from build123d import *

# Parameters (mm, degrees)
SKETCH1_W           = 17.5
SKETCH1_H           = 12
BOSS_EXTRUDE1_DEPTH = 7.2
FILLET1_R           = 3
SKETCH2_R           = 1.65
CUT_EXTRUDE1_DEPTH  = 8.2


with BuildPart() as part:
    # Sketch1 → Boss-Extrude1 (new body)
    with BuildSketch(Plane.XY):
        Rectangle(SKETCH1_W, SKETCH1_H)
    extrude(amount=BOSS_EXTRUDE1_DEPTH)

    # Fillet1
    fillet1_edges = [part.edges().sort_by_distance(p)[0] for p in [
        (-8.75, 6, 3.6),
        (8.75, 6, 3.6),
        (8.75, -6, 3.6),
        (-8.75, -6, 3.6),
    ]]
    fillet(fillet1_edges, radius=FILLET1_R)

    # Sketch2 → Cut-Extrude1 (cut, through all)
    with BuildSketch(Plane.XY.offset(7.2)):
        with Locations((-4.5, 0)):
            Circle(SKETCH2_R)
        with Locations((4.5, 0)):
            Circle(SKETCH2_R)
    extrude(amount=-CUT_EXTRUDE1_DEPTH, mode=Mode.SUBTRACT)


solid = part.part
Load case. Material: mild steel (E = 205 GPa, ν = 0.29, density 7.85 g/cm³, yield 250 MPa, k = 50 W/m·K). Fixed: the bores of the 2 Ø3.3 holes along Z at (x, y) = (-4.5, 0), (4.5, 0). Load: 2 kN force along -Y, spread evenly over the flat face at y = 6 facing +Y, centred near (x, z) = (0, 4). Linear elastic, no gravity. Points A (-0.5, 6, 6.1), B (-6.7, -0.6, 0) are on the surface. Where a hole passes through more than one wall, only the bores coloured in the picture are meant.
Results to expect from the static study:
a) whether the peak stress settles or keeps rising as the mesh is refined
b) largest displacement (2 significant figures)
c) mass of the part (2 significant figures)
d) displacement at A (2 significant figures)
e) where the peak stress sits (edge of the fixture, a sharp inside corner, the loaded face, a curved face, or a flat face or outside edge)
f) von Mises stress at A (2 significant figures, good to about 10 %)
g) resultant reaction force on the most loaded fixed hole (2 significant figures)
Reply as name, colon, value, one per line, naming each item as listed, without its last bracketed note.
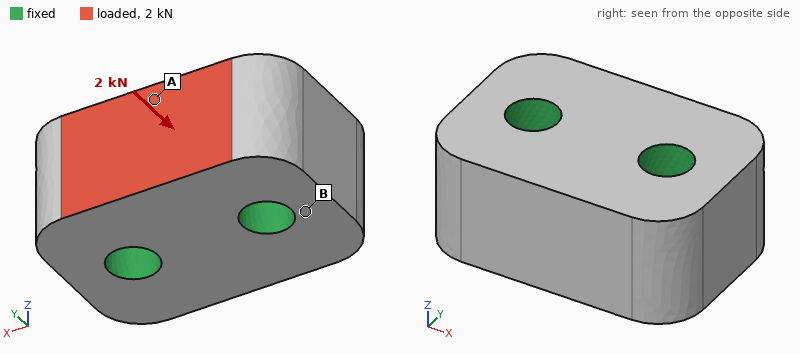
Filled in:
whether the peak stress settles or keeps rising as the mesh is refined: keeps rising
largest displacement: 0.75 µm
mass of the part: 10 g
displacement at A: 0.71 µm
where the peak stress sits: edge of the fixture
von Mises stress at A: 21 MPa
resultant reaction force on the most loaded fixed hole: 1.0 kN
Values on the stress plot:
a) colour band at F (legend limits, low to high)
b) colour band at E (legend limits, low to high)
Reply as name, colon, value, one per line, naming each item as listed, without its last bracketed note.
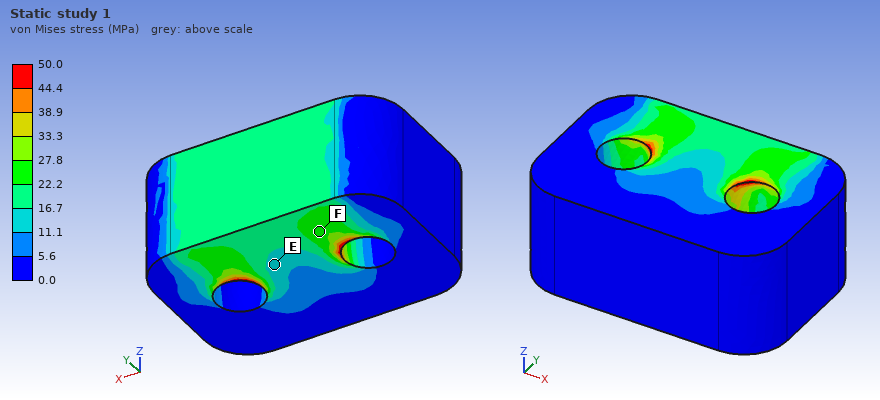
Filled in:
colour band at F: 22.2 to 27.8 MPa
colour band at E: 11.1 to 16.7 MPa
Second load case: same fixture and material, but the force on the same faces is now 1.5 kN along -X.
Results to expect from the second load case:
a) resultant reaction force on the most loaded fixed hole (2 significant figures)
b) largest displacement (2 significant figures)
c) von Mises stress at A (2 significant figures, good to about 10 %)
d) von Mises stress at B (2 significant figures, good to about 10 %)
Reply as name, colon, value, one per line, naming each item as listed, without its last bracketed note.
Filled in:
resultant reaction force on the most loaded fixed hole: 1.0 kN
largest displacement: 1.2 µm
von Mises stress at A: 31 MPa
von Mises stress at B: 14 MPa
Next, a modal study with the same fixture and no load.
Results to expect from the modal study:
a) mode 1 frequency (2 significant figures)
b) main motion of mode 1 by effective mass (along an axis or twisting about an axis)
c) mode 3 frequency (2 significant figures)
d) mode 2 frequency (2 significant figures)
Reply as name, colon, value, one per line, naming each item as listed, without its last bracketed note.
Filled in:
mode 1 frequency: 110 kHz
main motion of mode 1 by effective mass: twisting about X
mode 3 frequency: 120 kHz
mode 2 frequency: 120 kHz
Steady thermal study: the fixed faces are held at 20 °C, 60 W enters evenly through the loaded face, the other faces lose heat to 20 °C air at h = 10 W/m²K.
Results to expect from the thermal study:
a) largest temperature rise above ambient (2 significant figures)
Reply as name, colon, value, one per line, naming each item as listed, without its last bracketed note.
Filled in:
largest temperature rise above ambient: 69 K
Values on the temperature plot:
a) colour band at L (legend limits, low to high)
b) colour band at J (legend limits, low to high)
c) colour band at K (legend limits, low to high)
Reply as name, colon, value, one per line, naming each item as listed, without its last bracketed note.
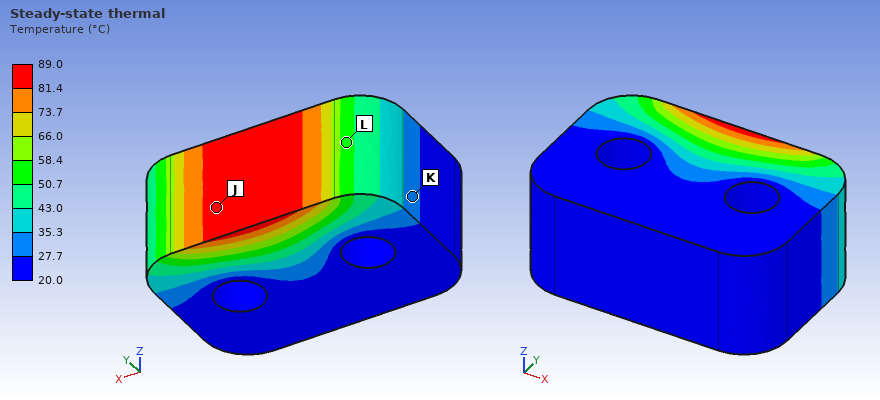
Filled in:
colour band at L: 50.7 to 58.4 °C
colour band at J: 81.4 to 89.0 °C
colour band at K: 27.7 to 35.3 °C
